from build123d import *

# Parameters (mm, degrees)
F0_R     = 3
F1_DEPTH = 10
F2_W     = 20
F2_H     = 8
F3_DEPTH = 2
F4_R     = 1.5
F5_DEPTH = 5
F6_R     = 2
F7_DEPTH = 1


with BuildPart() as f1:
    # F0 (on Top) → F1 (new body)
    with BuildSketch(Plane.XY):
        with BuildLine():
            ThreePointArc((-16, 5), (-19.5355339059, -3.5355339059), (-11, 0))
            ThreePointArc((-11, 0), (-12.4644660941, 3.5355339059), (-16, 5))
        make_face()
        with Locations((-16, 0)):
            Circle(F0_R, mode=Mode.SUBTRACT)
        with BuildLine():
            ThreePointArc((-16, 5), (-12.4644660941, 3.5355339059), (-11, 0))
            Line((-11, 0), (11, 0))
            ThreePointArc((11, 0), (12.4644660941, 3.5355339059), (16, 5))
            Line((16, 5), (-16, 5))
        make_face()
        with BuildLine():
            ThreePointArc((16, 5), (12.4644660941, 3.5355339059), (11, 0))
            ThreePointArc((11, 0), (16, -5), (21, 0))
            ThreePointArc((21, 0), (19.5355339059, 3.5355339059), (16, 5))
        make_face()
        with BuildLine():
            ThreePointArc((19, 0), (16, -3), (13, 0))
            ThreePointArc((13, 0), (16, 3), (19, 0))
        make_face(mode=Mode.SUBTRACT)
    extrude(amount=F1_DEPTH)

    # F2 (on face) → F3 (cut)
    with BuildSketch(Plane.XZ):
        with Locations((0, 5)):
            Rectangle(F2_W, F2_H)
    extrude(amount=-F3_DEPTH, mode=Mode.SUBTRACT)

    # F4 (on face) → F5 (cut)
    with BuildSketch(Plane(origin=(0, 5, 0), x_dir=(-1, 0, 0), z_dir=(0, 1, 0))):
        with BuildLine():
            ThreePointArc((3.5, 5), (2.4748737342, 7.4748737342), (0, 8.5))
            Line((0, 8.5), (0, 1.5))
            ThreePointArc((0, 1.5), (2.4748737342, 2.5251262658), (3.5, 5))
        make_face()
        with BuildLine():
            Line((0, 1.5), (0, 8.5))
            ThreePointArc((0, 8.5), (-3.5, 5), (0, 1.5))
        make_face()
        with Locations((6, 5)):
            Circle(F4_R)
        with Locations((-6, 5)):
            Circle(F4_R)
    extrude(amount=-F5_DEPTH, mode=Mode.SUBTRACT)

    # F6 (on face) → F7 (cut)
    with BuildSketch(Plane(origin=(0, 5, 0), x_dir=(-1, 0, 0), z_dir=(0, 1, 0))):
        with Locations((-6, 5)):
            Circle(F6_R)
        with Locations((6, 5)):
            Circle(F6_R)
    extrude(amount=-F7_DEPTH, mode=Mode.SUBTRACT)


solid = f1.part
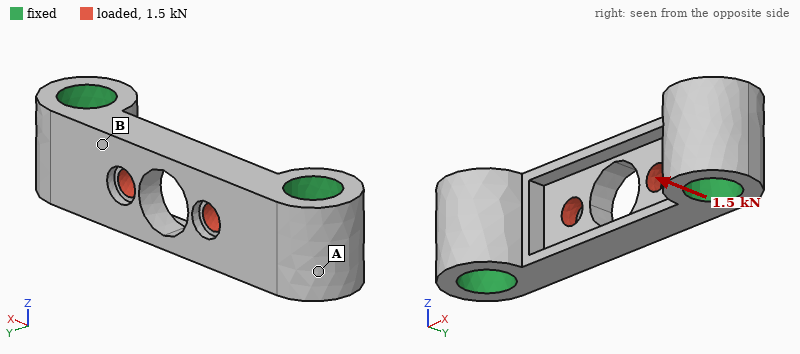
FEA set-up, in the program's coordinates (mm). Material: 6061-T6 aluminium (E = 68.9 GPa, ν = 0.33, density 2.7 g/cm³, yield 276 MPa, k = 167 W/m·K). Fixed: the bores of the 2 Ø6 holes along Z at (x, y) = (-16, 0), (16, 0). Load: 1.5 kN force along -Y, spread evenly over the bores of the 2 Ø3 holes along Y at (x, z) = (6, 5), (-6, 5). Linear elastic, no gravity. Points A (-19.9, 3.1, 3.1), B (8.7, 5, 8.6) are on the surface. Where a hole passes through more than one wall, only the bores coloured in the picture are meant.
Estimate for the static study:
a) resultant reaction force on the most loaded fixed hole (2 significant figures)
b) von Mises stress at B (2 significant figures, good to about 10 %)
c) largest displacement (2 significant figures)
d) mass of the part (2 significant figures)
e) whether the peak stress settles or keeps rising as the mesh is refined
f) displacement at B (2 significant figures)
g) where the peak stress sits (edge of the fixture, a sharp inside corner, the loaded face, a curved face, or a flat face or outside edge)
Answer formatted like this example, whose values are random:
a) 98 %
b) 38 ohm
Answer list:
a) 760 N
b) 65 MPa
c) 36 µm
d) 4.7 g
e) keeps rising
f) 11 µm
g) a sharp inside corner
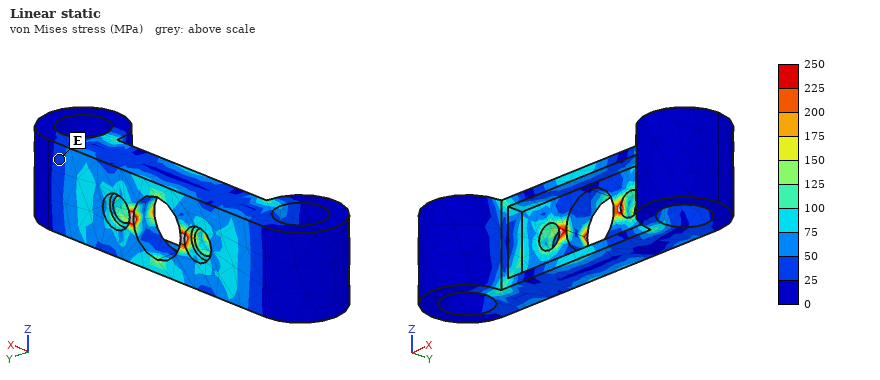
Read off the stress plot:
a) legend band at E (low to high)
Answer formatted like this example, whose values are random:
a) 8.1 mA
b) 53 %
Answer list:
a) 25 to 50 MPa
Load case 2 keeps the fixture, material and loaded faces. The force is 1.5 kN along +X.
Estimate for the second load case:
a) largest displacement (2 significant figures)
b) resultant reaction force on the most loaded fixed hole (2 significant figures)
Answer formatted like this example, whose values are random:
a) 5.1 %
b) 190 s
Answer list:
a) 7.8 µm
b) 750 N
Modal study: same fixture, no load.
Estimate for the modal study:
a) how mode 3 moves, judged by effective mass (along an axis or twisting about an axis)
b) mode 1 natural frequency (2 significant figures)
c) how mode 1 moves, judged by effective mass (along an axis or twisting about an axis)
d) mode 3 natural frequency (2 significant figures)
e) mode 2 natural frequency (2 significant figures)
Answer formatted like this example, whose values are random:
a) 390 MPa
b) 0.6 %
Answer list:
a) along Z
b) 34 kHz
c) along Y
d) 47 kHz
e) 37 kHz
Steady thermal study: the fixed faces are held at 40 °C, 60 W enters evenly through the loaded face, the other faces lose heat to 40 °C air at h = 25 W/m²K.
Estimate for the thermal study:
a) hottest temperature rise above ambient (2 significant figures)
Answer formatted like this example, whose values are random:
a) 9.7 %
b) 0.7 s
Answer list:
a) 54 K
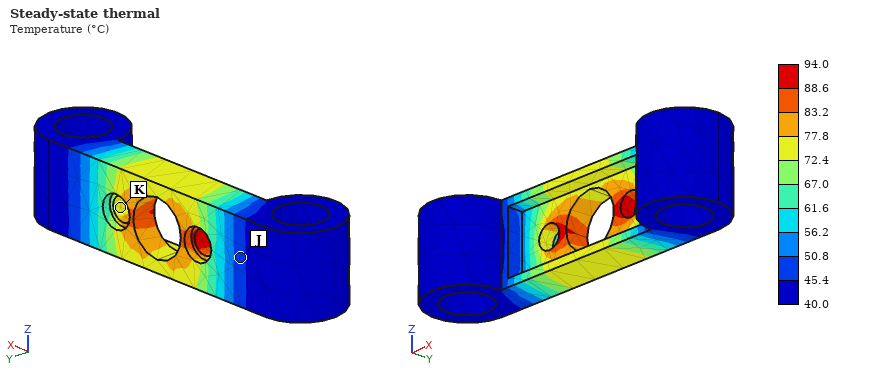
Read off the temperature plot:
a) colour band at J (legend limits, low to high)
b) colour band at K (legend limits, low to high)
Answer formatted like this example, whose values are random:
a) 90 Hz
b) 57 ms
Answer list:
a) 45.4 to 50.8 °C
b) 72.4 to 77.8 °C
